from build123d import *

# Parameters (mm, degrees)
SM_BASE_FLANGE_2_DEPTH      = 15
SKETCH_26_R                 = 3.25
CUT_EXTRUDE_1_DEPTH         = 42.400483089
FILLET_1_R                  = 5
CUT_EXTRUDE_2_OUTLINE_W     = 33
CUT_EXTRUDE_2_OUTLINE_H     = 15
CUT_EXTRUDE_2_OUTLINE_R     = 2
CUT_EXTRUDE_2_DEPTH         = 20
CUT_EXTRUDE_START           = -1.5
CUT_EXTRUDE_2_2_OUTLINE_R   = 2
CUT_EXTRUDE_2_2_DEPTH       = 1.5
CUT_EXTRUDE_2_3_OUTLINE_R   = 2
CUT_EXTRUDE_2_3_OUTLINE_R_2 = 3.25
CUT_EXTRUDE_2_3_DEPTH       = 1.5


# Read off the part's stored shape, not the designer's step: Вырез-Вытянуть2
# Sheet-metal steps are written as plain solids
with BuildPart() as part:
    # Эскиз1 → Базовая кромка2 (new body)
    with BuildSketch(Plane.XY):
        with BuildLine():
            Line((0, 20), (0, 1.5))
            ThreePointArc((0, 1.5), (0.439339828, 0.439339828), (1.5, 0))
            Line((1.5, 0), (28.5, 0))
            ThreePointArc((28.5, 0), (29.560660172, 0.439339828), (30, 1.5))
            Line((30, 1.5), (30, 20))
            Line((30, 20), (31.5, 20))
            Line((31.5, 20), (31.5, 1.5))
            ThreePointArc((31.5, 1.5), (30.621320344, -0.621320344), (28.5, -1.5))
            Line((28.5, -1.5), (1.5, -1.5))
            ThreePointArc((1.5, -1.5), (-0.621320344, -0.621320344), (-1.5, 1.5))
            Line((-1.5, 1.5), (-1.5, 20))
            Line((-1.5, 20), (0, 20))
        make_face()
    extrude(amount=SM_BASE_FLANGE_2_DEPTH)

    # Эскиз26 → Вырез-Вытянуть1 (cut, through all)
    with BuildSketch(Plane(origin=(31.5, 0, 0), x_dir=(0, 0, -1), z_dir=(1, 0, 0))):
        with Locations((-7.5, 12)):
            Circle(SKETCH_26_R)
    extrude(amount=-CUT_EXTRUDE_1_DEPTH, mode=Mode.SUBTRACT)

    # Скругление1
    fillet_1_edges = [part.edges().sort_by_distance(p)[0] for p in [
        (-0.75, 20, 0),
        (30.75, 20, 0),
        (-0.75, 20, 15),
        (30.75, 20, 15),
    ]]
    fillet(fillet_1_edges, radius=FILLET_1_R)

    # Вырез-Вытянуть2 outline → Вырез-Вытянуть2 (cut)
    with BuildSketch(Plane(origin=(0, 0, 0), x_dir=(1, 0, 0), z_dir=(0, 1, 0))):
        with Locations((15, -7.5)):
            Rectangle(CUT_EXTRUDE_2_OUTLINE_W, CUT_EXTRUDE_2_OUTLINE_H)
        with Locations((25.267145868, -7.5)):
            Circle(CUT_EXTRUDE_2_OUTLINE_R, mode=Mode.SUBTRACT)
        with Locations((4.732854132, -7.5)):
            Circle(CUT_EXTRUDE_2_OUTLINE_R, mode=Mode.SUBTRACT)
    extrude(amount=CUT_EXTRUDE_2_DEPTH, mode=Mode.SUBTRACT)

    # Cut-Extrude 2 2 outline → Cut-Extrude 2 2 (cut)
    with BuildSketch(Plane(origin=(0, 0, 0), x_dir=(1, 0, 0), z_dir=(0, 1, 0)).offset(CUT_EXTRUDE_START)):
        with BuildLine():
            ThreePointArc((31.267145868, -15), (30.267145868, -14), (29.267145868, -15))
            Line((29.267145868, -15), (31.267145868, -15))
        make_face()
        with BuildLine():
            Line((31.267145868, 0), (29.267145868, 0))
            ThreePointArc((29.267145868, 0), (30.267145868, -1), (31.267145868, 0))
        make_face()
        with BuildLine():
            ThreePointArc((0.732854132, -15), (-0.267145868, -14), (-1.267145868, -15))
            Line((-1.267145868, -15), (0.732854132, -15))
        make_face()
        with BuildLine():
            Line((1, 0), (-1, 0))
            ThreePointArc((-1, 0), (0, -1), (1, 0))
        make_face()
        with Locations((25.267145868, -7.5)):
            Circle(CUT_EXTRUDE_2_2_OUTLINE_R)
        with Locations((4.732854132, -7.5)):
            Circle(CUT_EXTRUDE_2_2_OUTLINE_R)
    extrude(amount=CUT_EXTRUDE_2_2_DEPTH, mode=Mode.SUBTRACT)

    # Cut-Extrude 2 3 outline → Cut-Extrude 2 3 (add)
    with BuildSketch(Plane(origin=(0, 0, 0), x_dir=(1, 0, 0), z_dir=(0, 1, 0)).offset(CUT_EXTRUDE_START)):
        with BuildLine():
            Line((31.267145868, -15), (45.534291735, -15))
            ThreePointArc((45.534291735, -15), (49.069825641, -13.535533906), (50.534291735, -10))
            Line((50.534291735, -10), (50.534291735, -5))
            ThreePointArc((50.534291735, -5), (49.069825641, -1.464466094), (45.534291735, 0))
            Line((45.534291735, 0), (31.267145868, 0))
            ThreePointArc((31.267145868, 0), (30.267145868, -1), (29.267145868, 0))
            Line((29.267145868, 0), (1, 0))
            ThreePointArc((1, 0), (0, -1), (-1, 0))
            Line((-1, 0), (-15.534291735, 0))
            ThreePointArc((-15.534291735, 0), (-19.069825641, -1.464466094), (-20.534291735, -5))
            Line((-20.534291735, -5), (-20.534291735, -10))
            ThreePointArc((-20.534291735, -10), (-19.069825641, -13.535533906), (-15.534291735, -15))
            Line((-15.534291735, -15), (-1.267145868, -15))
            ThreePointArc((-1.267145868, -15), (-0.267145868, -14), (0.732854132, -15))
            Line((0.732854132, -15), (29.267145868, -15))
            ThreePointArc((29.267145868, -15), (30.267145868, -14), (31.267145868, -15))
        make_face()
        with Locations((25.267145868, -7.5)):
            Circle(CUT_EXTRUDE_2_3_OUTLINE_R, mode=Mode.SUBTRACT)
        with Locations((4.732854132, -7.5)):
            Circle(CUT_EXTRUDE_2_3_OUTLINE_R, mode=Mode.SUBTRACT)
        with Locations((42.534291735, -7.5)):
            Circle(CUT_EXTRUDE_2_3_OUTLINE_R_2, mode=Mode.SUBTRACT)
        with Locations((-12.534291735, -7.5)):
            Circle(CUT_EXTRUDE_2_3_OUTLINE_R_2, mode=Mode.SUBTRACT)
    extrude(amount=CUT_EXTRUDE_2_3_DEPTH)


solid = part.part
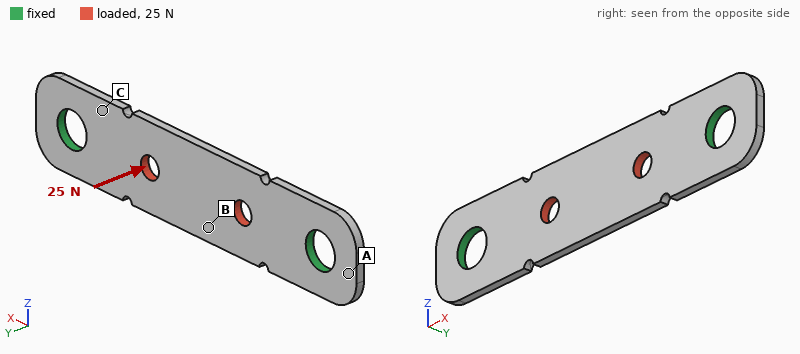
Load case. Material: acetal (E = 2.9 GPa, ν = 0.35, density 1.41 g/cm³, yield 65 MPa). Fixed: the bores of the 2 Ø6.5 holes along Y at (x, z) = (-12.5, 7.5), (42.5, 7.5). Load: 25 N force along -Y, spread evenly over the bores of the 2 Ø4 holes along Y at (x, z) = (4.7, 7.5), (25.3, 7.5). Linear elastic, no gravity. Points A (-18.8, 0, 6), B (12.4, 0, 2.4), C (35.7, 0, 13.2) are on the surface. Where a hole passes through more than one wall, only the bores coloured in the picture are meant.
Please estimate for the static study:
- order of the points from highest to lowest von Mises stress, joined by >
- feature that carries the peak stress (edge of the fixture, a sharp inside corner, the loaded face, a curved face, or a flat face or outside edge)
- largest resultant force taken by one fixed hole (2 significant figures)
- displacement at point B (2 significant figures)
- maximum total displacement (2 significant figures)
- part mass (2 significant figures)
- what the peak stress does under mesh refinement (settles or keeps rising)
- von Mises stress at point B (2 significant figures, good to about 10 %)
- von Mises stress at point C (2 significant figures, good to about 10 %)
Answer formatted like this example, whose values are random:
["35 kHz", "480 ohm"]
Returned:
["C > B > A", "edge of the fixture", "13 N", "0.82 mm", "0.85 mm", "2.0 g", "keeps rising", "9.0 MPa", "13 MPa"]
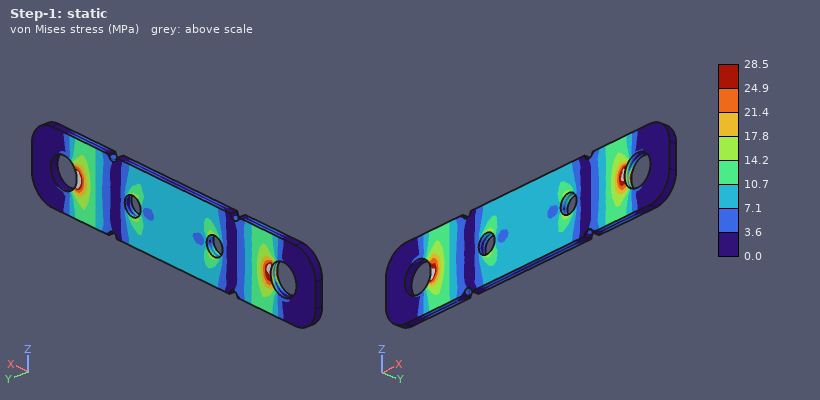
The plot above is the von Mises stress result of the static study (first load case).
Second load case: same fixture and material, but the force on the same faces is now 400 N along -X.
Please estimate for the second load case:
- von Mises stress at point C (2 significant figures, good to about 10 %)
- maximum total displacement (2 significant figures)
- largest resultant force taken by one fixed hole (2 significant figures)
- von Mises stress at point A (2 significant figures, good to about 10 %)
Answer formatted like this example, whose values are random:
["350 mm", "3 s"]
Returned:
["7.0 MPa", "72 µm", "200 N", "1.6 MPa"]
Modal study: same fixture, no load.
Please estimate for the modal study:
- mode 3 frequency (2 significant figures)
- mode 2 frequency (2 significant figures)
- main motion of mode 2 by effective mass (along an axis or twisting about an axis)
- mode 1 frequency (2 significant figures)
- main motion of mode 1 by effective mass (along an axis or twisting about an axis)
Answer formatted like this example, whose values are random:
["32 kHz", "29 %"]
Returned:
["2400 Hz", "1800 Hz", "twisting about X", "900 Hz", "along Y"]
